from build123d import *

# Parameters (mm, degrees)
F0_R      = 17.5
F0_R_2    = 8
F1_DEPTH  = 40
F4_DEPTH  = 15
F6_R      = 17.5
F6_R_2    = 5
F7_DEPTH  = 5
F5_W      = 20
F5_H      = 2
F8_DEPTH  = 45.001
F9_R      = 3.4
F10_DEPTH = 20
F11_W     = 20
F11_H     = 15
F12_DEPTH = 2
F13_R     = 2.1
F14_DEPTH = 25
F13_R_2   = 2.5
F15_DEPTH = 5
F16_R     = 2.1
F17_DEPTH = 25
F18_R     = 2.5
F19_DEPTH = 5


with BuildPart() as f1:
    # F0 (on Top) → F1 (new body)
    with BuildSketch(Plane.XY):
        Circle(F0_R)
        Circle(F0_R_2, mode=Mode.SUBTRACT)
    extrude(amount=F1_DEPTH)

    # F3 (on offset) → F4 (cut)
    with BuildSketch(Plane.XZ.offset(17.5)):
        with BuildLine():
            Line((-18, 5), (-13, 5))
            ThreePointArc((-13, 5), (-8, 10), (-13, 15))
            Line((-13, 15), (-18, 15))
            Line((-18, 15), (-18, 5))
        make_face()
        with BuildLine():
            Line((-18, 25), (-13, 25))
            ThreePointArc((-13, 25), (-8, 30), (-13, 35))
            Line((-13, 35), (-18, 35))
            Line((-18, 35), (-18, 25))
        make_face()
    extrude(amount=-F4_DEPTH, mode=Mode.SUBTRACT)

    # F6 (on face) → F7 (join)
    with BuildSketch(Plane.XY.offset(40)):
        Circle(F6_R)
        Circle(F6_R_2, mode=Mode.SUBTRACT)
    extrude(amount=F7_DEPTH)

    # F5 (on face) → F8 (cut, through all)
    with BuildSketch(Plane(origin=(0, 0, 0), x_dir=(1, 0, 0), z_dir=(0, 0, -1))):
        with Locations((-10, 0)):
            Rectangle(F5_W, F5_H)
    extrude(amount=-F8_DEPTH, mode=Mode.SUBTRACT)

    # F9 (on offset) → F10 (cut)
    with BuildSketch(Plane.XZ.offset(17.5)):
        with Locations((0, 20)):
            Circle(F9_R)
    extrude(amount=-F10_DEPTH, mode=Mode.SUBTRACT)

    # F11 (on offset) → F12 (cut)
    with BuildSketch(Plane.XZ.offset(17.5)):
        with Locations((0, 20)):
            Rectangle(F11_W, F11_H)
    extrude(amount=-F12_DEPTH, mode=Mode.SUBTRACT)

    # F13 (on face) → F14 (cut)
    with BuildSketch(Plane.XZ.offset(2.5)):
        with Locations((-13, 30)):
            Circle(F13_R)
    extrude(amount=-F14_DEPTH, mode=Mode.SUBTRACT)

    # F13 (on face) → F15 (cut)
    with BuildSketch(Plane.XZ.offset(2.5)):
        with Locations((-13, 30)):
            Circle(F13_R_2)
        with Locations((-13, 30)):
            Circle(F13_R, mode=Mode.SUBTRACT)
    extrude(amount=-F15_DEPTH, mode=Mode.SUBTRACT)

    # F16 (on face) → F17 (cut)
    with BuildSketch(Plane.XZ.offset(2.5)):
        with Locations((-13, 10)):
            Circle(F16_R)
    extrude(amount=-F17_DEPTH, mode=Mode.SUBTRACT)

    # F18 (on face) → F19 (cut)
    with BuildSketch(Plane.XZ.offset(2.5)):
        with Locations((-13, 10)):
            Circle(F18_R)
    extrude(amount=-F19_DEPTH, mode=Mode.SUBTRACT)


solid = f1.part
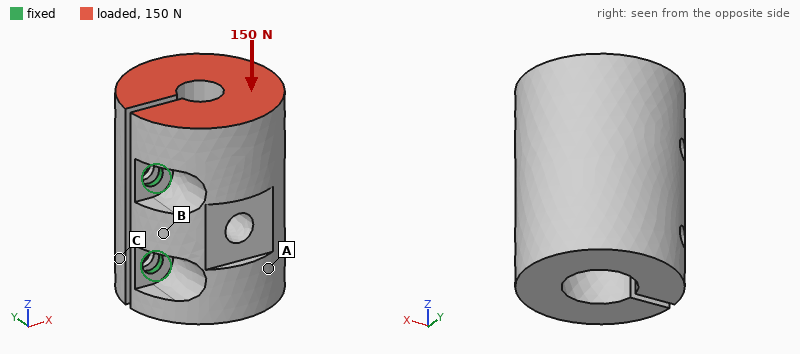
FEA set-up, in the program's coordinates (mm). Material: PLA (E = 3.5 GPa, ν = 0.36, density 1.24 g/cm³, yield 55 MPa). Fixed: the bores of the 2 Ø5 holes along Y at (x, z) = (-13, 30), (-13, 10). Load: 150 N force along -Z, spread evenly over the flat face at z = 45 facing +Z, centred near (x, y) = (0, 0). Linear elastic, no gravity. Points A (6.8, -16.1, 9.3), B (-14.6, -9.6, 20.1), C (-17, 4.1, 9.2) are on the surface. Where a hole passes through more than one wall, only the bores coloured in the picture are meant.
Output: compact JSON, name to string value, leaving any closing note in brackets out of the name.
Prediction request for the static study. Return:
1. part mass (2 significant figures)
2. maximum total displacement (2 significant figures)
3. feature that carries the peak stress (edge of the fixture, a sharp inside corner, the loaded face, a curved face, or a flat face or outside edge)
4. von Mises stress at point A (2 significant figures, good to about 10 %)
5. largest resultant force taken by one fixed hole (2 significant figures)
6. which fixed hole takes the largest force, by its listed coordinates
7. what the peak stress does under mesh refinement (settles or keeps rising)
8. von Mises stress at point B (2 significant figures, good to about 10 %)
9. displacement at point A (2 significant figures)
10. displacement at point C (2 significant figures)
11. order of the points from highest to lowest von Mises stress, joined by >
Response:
{"part mass": "39 g", "maximum total displacement": "0.21 mm", "feature that carries the peak stress": "edge of the fixture", "von Mises stress at point A": "2.0 MPa", "largest resultant force taken by one fixed hole": "110 N", "which fixed hole takes the largest force, by its listed coordinates": "(-13, 30)", "what the peak stress does under mesh refinement": "keeps rising", "von Mises stress at point B": "3.1 MPa", "displacement at point A": "0.070 mm", "displacement at point C": "0.11 mm", "order of the points from highest to lowest von Mises stress, joined by >": "B > A > C"}
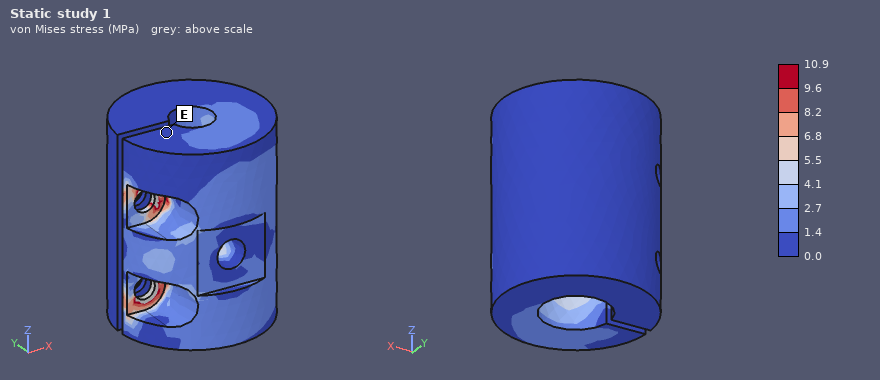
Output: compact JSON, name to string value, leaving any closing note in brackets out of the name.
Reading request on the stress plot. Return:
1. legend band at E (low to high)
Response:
{"legend band at E": "0.0 to 1.4 MPa"}
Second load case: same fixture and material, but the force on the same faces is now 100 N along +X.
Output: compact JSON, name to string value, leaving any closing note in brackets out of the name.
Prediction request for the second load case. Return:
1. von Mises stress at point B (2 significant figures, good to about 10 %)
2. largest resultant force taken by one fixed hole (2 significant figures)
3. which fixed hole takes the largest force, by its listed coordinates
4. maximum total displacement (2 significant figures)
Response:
{"von Mises stress at point B": "2.6 MPa", "largest resultant force taken by one fixed hole": "150 N", "which fixed hole takes the largest force, by its listed coordinates": "(-13, 30)", "maximum total displacement": "0.23 mm"}
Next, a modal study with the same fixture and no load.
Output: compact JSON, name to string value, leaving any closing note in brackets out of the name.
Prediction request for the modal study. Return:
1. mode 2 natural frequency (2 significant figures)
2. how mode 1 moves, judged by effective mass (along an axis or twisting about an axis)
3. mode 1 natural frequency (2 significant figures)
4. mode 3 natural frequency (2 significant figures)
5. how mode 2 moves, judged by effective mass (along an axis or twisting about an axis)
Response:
{"mode 2 natural frequency": "700 Hz", "how mode 1 moves, judged by effective mass": "along Y", "mode 1 natural frequency": "310 Hz", "mode 3 natural frequency": "1000 Hz", "how mode 2 moves, judged by effective mass": "along Z"}
